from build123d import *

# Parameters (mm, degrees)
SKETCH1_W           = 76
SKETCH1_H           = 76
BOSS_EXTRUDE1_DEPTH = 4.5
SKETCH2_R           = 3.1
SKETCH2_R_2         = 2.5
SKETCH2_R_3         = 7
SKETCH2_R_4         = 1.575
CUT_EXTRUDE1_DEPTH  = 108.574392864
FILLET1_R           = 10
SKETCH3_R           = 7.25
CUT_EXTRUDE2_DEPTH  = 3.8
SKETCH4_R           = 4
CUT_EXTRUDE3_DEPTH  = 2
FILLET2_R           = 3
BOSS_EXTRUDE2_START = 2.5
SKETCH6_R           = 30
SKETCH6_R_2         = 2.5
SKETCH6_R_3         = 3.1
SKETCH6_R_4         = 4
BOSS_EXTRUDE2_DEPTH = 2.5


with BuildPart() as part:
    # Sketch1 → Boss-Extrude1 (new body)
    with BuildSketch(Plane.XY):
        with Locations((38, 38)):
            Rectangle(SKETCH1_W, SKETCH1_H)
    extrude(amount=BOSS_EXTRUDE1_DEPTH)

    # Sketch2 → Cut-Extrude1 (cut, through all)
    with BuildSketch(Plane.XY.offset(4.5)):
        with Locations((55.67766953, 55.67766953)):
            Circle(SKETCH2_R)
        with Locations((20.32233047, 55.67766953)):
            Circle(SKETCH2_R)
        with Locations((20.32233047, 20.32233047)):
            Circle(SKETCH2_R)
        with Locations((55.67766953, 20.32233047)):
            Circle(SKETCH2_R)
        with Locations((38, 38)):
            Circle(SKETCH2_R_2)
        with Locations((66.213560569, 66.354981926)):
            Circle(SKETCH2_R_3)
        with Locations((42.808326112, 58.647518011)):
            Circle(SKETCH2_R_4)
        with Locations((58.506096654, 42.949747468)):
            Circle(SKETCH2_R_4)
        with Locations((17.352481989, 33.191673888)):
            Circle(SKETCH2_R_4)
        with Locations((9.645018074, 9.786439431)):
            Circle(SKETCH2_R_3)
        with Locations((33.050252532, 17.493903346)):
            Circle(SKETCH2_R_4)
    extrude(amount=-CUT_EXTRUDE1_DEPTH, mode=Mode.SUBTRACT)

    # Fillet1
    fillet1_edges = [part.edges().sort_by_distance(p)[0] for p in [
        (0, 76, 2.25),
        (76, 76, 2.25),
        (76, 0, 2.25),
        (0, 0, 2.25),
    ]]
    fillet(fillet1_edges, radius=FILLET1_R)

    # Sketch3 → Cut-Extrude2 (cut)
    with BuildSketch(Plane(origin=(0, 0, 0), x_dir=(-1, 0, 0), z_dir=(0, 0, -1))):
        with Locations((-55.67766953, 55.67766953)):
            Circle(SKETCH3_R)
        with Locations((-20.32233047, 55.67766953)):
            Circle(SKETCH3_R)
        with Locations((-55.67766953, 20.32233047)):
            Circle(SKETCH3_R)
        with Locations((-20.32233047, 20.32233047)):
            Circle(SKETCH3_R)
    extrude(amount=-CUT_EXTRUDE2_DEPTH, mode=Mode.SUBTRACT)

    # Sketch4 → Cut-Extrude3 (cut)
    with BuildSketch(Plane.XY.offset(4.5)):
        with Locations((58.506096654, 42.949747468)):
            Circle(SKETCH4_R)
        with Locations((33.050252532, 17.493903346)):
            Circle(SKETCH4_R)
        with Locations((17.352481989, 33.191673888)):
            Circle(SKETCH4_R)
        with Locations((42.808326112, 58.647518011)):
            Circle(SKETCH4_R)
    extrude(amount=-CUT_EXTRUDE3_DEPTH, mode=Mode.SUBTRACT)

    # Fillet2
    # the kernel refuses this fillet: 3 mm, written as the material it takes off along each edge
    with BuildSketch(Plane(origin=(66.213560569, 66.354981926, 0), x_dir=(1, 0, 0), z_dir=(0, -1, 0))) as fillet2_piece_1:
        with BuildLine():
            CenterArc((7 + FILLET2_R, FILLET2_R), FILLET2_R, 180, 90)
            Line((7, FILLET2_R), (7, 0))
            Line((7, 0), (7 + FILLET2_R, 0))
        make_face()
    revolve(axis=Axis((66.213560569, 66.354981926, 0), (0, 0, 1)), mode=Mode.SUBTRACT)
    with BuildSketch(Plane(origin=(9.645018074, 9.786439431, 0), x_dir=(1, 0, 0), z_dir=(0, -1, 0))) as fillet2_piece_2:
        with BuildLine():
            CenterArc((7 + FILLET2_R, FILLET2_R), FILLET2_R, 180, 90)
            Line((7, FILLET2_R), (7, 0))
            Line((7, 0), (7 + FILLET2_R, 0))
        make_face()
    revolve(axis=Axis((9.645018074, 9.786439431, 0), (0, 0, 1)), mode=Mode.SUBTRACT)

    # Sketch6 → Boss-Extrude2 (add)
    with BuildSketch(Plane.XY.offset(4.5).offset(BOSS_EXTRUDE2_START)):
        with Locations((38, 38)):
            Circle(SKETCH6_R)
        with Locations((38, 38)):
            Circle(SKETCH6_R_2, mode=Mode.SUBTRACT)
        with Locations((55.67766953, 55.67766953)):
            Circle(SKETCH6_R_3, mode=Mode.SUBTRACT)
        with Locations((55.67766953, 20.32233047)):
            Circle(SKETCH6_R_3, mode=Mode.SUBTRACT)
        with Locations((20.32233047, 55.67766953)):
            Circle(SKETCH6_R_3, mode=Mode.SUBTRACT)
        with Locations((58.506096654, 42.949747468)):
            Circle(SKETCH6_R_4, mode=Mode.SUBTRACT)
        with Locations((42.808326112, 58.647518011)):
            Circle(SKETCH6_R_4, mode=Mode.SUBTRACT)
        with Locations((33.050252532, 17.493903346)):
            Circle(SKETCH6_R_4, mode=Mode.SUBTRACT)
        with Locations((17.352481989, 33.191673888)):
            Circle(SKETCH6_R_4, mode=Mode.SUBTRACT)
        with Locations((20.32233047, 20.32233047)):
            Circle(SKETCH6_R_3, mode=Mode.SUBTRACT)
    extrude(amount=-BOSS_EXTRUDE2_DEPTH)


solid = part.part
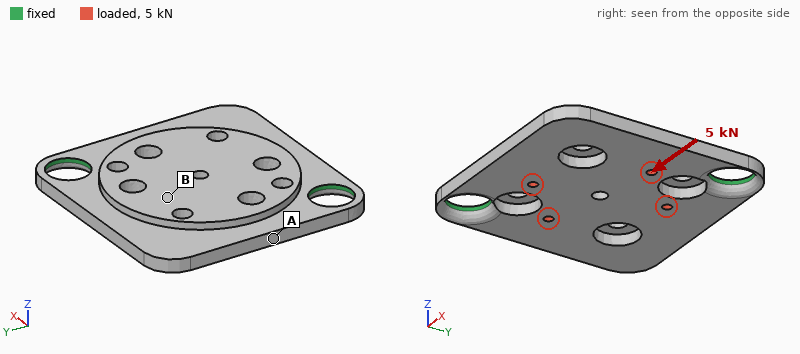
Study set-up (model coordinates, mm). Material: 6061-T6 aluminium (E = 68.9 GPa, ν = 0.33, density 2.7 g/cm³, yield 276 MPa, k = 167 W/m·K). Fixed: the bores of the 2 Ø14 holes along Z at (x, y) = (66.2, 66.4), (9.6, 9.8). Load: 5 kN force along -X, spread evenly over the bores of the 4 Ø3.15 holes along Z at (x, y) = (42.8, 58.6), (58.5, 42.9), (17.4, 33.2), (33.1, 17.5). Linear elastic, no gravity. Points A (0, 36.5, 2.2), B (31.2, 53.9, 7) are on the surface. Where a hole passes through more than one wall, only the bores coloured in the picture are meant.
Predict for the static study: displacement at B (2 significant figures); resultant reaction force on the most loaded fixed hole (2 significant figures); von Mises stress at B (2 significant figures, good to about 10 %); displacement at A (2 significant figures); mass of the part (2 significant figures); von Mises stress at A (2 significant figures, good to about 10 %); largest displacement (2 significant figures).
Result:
0.040 mm
2.5 kN
9.7 MPa
0.061 mm
73 g
22 MPa
0.12 mm
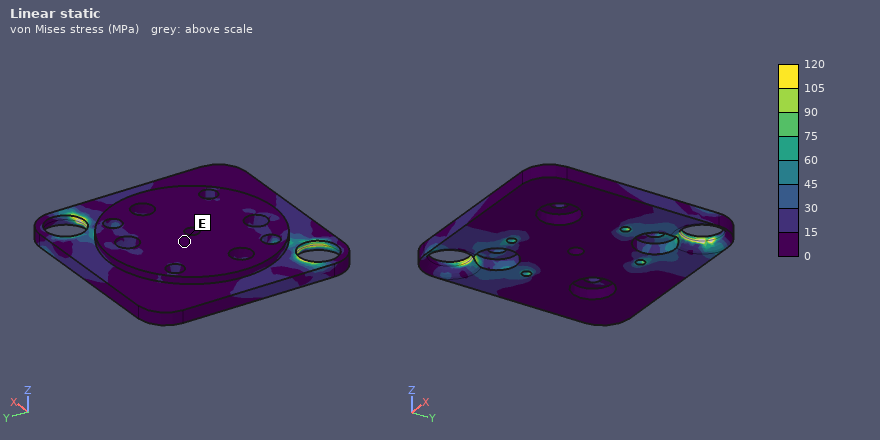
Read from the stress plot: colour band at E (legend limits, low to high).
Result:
0 to 15 MPa
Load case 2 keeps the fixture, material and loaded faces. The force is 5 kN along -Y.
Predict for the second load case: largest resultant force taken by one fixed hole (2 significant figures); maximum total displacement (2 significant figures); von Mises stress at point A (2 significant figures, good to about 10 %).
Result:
2.5 kN
0.12 mm
17 MPa
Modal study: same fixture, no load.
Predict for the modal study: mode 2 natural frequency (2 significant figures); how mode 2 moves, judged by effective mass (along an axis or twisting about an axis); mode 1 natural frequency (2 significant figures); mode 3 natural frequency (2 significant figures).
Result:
2200 Hz
along Z
1500 Hz
6300 Hz
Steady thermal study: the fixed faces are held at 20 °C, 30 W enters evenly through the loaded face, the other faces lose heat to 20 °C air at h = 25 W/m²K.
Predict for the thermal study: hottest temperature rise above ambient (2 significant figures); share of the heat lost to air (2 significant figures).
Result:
15 K
10 %
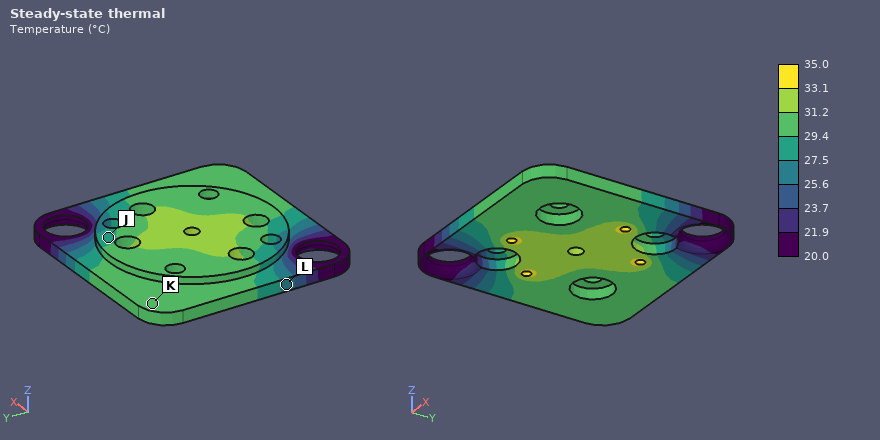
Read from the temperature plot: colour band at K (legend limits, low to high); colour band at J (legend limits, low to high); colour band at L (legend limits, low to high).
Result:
29.4 to 31.2 °C
27.5 to 29.4 °C
25.6 to 27.5 °C
